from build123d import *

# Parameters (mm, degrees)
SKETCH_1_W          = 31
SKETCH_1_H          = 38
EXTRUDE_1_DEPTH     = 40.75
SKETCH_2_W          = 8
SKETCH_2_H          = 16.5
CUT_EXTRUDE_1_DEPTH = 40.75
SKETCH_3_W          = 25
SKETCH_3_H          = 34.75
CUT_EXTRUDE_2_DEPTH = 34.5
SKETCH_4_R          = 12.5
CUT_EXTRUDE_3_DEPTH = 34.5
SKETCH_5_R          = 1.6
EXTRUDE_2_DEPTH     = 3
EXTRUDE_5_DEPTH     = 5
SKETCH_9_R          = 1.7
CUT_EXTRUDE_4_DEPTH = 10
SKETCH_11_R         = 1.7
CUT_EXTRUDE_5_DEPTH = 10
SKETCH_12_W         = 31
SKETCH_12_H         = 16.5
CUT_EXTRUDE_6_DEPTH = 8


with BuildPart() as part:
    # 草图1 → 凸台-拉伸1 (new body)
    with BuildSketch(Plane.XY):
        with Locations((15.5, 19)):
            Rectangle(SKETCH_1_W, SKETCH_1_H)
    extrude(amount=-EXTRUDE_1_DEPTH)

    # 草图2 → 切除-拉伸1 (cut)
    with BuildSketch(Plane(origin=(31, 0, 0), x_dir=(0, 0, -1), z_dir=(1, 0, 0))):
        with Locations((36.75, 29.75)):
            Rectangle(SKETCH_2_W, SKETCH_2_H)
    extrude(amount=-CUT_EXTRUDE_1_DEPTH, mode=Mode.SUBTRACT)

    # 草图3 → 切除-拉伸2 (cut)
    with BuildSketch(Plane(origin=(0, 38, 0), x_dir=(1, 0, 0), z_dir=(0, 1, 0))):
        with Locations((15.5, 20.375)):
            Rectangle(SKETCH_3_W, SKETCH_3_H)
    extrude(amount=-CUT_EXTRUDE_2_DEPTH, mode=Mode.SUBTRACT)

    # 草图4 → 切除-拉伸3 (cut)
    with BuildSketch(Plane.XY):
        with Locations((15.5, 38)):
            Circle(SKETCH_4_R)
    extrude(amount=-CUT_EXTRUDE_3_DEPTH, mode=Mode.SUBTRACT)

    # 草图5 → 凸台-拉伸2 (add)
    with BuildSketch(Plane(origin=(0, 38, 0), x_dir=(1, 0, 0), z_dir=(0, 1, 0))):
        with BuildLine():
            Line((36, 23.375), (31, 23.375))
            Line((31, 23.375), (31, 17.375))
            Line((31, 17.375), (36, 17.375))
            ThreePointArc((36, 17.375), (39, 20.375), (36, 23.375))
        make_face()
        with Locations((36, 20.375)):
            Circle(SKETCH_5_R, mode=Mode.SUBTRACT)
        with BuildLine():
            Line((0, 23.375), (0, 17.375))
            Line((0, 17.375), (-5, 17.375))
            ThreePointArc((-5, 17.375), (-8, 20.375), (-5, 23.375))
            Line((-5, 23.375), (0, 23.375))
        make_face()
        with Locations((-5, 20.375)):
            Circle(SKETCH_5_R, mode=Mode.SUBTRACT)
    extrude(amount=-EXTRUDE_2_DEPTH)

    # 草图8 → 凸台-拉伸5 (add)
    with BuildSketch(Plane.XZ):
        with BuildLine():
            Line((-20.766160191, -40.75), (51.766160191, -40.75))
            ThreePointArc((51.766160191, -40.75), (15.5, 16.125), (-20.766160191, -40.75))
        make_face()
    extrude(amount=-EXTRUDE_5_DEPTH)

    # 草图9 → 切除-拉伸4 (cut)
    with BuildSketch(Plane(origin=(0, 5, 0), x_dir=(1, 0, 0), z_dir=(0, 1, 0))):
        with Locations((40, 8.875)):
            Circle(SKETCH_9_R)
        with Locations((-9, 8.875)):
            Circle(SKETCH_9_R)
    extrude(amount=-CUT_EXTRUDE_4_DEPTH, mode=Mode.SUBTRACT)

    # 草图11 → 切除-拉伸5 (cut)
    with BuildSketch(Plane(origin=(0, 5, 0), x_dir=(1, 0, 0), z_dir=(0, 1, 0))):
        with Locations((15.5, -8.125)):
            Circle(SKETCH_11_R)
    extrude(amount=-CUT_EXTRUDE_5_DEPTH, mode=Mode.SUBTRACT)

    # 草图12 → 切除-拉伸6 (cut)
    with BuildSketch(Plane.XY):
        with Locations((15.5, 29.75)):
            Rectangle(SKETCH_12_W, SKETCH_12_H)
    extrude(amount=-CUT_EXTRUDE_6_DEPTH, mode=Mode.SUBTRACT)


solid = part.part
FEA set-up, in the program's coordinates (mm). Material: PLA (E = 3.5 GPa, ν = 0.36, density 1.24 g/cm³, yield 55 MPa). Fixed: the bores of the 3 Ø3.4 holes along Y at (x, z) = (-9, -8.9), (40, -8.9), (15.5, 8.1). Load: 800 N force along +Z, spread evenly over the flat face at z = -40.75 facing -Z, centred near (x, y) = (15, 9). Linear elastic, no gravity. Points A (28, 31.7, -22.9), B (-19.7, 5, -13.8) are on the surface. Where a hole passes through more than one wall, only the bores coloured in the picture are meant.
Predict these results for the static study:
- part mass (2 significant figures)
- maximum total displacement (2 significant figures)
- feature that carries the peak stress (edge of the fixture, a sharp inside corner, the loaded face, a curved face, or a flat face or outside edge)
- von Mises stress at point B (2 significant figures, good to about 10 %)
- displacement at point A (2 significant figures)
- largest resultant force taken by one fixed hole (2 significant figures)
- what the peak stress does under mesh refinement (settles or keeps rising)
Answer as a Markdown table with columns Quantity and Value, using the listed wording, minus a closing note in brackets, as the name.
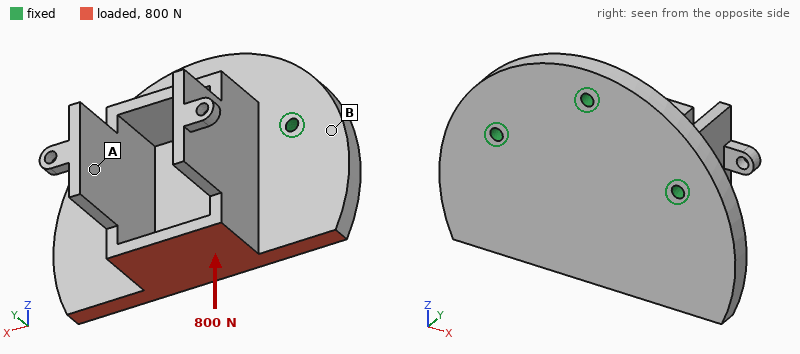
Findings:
| Quantity | Value |
|---|---|
| part mass | 35 g |
| maximum total displacement | 0.62 mm |
| feature that carries the peak stress | edge of the fixture |
| von Mises stress at point B | 3.9 MPa |
| displacement at point A | 0.36 mm |
| largest resultant force taken by one fixed hole | 300 N |
| what the peak stress does under mesh refinement | keeps rising |
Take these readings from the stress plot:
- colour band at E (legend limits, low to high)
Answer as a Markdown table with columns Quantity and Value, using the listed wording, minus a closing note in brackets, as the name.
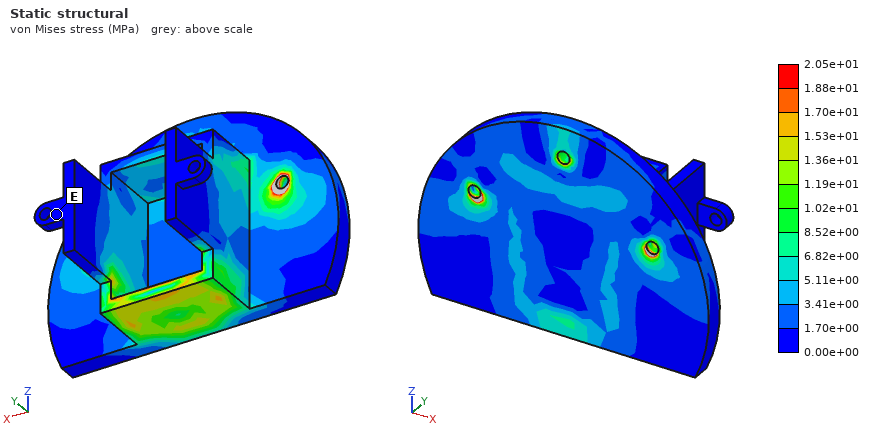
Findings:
| Quantity | Value |
|---|---|
| colour band at E | 0.00e+00 to 1.70e+00 MPa |
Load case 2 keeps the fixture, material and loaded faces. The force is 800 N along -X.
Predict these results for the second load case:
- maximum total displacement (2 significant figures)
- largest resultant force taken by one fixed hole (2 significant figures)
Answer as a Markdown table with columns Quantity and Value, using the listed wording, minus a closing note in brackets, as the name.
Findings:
| Quantity | Value |
|---|---|
| maximum total displacement | 0.54 mm |
| largest resultant force taken by one fixed hole | 650 N |
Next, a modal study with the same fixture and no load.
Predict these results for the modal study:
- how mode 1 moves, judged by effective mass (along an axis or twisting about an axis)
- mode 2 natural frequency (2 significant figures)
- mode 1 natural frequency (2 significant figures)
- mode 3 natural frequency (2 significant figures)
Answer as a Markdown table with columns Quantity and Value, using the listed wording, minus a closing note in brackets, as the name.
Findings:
| Quantity | Value |
|---|---|
| how mode 1 moves, judged by effective mass | along Y |
| mode 2 natural frequency | 1100 Hz |
| mode 1 natural frequency | 980 Hz |
| mode 3 natural frequency | 1100 Hz |
